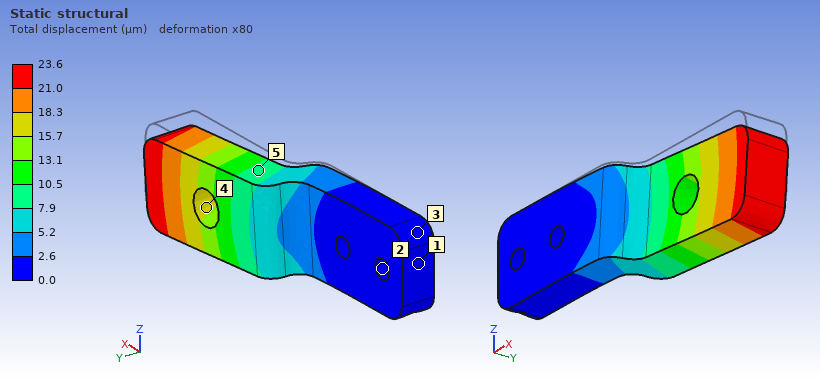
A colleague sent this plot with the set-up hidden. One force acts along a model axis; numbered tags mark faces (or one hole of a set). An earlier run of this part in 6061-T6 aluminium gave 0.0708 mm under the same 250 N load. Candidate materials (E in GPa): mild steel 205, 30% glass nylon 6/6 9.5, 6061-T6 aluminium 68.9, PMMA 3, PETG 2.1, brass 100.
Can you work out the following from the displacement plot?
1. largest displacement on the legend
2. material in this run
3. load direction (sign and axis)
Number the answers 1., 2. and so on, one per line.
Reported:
1. 23.6 µm
2. mild steel
3. -Z
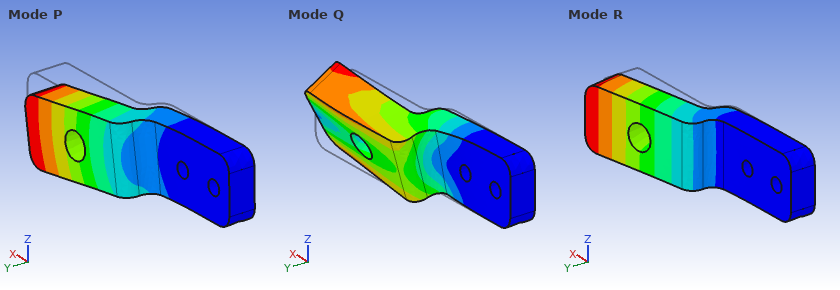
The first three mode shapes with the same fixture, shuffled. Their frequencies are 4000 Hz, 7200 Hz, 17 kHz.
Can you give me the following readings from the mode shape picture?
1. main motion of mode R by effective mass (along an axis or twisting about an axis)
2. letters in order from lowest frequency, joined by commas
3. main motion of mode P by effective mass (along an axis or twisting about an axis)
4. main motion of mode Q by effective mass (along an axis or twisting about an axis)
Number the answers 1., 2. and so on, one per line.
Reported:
1. along Y
2. R, P, Q
3. along Z
4. twisting about X
